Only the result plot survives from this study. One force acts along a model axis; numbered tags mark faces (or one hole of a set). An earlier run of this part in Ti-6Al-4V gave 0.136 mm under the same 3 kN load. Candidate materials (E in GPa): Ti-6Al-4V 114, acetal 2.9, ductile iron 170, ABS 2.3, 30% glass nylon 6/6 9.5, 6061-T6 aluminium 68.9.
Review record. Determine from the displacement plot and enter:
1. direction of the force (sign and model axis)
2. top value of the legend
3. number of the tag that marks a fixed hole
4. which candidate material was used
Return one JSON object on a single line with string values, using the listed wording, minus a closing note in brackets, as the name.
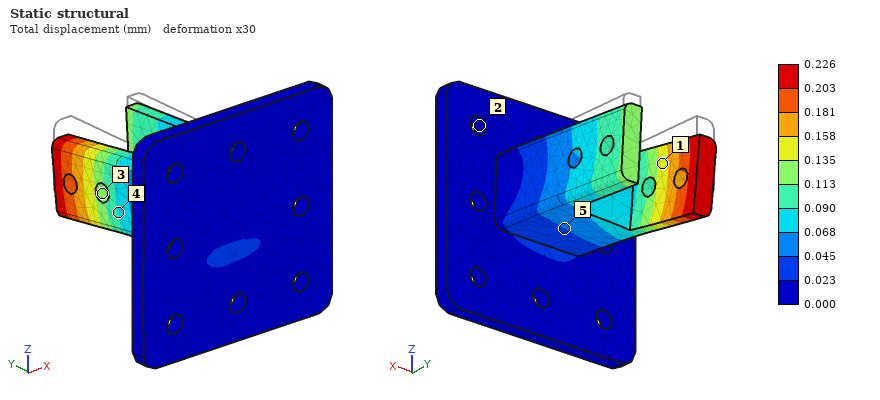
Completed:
{"direction of the force": "-Z", "top value of the legend": "0.226 mm", "number of the tag that marks a fixed hole": "2", "which candidate material was used": "6061-T6 aluminium"}
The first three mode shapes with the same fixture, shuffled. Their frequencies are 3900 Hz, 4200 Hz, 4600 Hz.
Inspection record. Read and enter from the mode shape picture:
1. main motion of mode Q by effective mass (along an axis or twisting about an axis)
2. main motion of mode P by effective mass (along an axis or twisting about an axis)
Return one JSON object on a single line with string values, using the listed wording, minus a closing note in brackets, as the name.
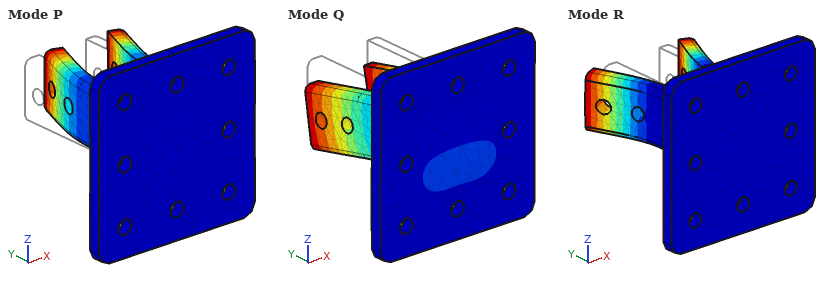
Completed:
{"main motion of mode Q by effective mass": "along Z", "main motion of mode P by effective mass": "along X"}
